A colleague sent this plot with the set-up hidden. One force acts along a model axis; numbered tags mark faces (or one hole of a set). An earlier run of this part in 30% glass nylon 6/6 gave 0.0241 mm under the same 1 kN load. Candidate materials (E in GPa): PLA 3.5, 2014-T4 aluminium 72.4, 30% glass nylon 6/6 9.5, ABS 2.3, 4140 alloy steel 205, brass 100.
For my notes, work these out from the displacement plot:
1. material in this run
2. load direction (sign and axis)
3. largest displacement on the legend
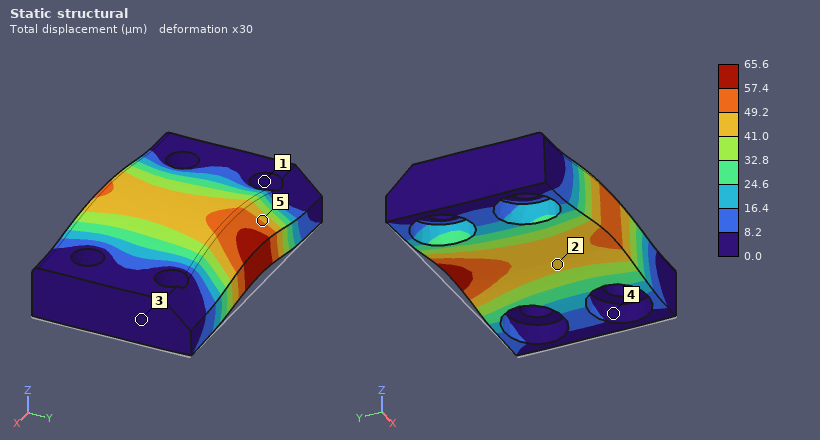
PLA
+Z
65.6 µm
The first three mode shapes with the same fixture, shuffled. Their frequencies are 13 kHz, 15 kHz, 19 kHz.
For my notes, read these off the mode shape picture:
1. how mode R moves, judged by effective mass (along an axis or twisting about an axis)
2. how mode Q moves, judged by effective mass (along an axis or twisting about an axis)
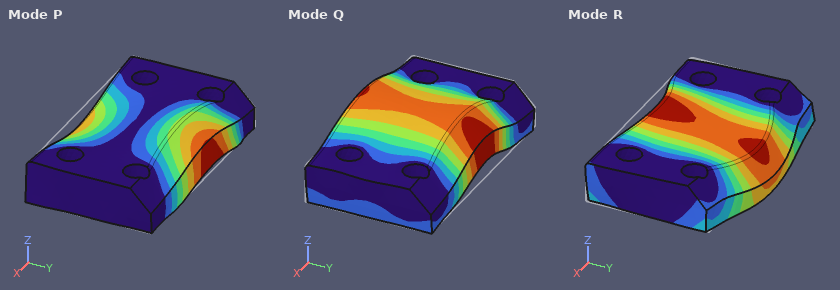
along Y
along Z
